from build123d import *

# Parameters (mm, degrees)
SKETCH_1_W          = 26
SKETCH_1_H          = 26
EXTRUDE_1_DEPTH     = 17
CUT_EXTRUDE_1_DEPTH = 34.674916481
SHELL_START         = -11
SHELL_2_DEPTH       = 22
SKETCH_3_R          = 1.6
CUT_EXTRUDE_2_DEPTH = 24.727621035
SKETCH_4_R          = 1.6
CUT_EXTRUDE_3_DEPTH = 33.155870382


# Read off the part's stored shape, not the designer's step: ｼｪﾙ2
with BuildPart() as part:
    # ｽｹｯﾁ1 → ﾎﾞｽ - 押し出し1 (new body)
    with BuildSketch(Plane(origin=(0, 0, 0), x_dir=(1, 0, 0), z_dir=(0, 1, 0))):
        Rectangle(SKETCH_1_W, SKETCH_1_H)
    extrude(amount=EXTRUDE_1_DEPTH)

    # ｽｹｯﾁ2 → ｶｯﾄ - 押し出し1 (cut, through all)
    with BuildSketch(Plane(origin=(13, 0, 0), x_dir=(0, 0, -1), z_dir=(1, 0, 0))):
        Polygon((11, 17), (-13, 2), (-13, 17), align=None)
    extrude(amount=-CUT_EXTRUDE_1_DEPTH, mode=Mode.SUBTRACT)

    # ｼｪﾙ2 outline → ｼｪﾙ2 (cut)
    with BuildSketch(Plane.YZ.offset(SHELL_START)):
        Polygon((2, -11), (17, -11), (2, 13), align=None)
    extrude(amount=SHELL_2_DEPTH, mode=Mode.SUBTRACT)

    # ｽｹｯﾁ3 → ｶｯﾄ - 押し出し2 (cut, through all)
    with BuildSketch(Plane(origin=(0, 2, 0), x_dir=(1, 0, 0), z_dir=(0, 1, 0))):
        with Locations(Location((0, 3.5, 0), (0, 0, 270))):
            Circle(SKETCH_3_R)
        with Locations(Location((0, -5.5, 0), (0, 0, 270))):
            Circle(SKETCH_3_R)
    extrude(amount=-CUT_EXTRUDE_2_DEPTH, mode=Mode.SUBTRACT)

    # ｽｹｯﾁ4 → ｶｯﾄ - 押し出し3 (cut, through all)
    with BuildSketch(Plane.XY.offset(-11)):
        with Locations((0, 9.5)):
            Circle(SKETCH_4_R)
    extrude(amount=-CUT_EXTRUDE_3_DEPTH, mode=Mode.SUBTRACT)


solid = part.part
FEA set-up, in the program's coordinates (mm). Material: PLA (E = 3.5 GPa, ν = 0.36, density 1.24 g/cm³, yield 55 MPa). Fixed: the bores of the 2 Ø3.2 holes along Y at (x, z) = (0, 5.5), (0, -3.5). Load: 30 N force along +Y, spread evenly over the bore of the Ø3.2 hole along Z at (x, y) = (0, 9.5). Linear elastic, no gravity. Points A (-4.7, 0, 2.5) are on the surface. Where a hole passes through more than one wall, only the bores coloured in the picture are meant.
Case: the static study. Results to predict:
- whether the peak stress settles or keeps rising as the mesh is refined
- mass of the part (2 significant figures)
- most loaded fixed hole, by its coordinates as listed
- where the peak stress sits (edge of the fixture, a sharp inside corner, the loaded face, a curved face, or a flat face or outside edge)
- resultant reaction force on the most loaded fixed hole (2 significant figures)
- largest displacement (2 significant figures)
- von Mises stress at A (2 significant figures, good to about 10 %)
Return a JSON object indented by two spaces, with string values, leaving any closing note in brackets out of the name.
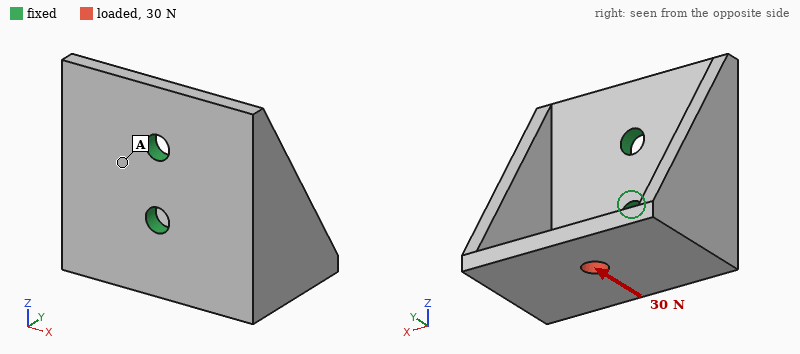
{
  "whether the peak stress settles or keeps rising as the mesh is refined": "keeps rising",
  "mass of the part": "3.5 g",
  "most loaded fixed hole, by its coordinates as listed": "(0, -3.5)",
  "where the peak stress sits": "edge of the fixture",
  "resultant reaction force on the most loaded fixed hole": "41 N",
  "largest displacement": "0.13 mm",
  "von Mises stress at A": "2.2 MPa"
}
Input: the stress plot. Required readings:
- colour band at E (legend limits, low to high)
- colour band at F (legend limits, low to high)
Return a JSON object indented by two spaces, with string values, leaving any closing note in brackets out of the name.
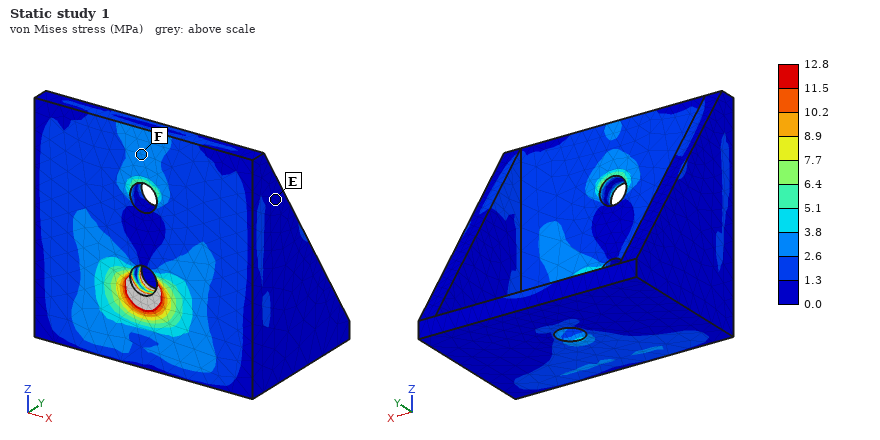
{
  "colour band at E": "0.0 to 1.3 MPa",
  "colour band at F": "2.6 to 3.8 MPa"
}
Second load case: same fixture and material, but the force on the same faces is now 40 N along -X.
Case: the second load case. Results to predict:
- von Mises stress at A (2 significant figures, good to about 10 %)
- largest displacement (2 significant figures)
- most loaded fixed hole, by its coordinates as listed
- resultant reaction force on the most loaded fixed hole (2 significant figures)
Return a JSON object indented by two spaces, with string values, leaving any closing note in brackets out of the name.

{
  "von Mises stress at A": "7.1 MPa",
  "largest displacement": "0.42 mm",
  "most loaded fixed hole, by its coordinates as listed": "(0, -3.5)",
  "resultant reaction force on the most loaded fixed hole": "65 N"
}
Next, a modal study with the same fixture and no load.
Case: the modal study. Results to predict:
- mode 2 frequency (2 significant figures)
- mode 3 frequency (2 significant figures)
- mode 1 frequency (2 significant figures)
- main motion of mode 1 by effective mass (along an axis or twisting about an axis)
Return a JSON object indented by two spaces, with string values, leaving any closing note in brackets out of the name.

{
  "mode 2 frequency": "1900 Hz",
  "mode 3 frequency": "2900 Hz",
  "mode 1 frequency": "1200 Hz",
  "main motion of mode 1 by effective mass": "along X"
}
